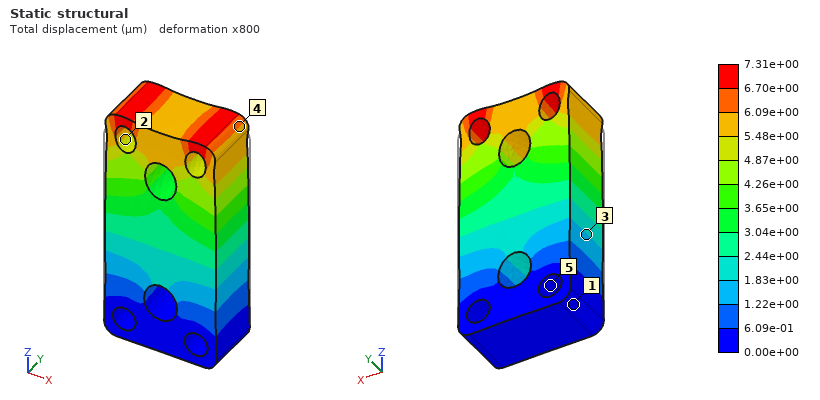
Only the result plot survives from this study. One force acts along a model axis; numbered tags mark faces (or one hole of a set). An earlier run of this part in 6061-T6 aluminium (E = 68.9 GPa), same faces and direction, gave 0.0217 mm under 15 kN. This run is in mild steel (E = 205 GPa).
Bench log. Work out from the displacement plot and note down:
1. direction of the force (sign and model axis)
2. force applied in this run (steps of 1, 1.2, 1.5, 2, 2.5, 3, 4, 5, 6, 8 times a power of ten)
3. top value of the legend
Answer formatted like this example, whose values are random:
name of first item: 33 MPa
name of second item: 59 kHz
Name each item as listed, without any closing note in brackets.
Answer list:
direction of the force: +Z
force applied in this run: 15 kN
top value of the legend: 7.31e+00 µm
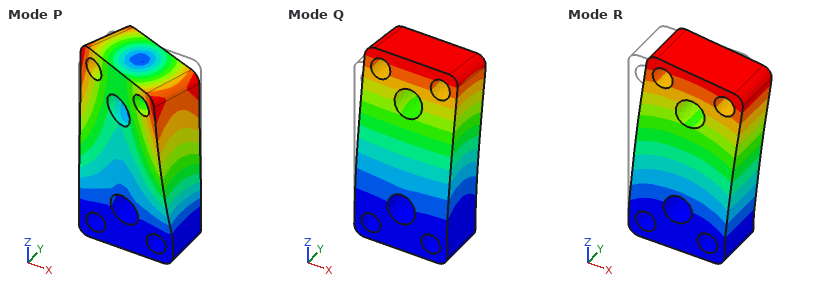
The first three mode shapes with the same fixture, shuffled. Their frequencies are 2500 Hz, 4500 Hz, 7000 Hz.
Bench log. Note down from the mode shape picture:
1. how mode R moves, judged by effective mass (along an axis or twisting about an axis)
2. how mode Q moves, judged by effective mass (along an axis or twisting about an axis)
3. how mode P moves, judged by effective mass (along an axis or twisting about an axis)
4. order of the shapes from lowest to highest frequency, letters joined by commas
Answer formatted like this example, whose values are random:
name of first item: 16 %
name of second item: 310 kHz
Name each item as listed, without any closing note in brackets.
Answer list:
how mode R moves, judged by effective mass: along X
how mode Q moves, judged by effective mass: along Y
how mode P moves, judged by effective mass: twisting about Z
order of the shapes from lowest to highest frequency, letters joined by commas: Q, R, P
